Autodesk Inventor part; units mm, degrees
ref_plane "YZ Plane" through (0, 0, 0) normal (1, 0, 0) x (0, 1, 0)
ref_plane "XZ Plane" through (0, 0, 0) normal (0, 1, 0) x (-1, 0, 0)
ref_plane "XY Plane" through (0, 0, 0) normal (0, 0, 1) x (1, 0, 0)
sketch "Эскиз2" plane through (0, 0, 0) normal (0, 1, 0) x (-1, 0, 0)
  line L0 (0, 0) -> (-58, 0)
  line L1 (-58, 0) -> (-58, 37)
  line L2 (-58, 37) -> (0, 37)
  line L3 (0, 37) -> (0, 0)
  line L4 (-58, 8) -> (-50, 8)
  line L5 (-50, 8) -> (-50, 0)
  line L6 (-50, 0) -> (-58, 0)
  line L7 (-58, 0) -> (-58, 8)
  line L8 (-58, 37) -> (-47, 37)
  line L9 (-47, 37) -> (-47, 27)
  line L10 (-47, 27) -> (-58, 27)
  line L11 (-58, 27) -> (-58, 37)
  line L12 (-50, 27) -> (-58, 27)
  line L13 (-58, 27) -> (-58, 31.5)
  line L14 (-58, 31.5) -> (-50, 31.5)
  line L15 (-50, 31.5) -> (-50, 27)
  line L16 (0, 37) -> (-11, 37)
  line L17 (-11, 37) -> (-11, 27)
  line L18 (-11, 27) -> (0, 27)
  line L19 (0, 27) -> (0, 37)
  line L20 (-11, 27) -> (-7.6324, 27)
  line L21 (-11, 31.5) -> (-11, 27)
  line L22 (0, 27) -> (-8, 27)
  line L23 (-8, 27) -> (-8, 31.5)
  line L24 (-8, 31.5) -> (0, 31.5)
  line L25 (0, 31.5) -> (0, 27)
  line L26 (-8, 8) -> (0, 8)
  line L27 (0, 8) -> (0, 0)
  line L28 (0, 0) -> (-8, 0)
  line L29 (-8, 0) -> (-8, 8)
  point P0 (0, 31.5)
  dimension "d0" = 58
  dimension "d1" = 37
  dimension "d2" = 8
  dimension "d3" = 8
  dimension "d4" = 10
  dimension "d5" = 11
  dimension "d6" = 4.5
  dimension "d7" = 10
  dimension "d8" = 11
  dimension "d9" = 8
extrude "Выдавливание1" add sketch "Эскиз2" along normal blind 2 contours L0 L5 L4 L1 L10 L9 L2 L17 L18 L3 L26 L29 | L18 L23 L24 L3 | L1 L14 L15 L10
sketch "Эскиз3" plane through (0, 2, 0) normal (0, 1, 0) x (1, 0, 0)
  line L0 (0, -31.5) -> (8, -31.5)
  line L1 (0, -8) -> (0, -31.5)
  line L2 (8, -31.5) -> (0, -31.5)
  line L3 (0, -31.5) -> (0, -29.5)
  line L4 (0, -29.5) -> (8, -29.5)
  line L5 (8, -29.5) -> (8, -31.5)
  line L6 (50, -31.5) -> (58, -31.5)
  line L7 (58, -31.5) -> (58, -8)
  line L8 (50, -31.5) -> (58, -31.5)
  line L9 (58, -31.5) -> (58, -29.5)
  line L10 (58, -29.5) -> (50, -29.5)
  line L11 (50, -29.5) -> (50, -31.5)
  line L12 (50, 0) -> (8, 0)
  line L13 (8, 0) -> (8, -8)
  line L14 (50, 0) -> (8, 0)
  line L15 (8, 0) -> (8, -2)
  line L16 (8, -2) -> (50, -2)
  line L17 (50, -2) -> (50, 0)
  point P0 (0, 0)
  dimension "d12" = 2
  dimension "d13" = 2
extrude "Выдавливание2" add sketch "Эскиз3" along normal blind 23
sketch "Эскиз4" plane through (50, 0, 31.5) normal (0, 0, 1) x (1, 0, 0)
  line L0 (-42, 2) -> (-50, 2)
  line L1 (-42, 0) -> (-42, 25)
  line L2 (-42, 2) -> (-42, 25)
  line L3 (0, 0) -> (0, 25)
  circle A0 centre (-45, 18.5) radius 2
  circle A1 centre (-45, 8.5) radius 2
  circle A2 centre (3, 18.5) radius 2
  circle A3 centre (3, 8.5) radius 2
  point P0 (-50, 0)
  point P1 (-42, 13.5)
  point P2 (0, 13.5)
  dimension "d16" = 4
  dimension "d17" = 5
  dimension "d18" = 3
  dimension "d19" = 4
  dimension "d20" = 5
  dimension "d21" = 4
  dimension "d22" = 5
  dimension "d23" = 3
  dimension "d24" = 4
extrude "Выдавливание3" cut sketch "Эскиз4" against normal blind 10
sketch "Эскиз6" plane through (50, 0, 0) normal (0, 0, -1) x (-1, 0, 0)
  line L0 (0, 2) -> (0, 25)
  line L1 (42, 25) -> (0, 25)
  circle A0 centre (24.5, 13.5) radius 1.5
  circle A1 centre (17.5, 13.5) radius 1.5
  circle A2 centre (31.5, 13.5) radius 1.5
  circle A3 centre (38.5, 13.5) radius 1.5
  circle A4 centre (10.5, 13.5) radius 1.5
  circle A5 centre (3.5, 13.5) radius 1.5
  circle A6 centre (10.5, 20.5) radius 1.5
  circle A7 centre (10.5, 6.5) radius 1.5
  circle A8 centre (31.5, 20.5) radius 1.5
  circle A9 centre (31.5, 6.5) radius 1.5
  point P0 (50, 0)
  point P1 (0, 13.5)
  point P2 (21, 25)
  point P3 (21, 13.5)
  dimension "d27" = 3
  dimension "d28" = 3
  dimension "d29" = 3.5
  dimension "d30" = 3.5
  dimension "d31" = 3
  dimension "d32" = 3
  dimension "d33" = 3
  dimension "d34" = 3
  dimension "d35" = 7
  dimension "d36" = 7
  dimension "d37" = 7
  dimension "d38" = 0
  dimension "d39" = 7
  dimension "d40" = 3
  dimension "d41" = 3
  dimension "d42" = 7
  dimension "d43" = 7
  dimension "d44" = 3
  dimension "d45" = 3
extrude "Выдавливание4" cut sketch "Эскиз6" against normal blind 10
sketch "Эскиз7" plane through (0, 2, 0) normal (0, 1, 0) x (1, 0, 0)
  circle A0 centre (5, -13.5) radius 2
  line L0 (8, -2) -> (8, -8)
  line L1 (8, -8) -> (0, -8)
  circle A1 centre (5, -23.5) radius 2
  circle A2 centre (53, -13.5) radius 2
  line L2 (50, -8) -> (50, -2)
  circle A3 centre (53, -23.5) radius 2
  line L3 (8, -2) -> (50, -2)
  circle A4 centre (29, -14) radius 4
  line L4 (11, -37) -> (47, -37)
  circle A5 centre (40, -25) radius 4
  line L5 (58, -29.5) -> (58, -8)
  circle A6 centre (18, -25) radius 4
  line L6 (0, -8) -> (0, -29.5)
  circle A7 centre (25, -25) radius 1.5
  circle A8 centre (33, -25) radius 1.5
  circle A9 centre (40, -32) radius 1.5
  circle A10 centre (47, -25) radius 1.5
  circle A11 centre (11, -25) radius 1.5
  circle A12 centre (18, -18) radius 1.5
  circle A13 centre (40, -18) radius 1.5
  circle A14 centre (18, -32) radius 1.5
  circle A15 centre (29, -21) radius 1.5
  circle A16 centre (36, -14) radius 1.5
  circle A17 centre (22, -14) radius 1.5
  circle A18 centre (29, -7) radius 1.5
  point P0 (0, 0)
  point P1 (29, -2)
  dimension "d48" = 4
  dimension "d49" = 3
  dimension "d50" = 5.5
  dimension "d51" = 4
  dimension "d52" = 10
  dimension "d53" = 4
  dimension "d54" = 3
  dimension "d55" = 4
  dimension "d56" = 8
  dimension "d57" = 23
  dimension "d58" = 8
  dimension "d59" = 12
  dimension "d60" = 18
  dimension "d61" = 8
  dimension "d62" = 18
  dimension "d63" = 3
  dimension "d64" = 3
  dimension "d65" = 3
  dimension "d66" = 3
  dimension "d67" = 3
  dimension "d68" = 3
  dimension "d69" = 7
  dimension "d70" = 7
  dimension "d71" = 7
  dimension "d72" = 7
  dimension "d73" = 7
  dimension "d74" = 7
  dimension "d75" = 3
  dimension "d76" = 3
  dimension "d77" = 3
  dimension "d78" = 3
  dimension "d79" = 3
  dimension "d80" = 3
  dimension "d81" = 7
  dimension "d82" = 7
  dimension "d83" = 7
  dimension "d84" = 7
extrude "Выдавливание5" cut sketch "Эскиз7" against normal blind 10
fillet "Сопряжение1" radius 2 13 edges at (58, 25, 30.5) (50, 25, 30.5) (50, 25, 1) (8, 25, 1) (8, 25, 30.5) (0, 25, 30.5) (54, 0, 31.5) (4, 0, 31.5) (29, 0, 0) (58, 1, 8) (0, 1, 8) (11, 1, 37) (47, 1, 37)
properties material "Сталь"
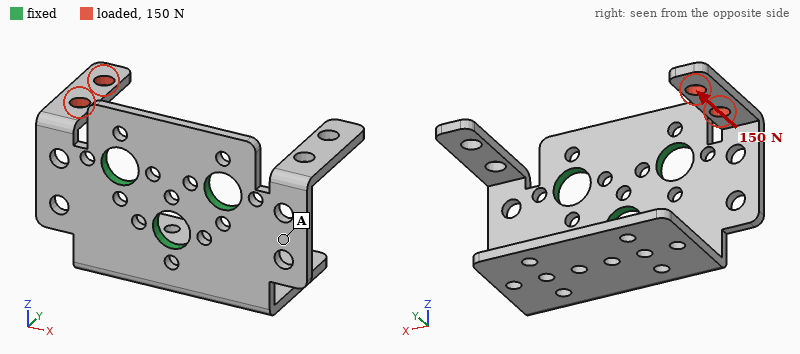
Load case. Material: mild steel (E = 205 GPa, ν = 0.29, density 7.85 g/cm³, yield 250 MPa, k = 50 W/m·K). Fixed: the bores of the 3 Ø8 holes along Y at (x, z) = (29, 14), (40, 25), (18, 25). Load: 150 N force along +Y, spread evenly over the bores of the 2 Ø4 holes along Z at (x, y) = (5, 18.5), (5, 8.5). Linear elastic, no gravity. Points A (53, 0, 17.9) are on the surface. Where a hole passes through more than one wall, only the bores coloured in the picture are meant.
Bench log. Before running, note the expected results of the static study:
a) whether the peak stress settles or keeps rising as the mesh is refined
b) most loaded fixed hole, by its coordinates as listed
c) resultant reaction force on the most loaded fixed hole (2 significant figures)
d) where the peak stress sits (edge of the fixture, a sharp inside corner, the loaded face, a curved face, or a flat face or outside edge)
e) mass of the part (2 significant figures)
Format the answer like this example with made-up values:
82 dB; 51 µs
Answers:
keeps rising; (18, 25); 180 N; a sharp inside corner; 43 g
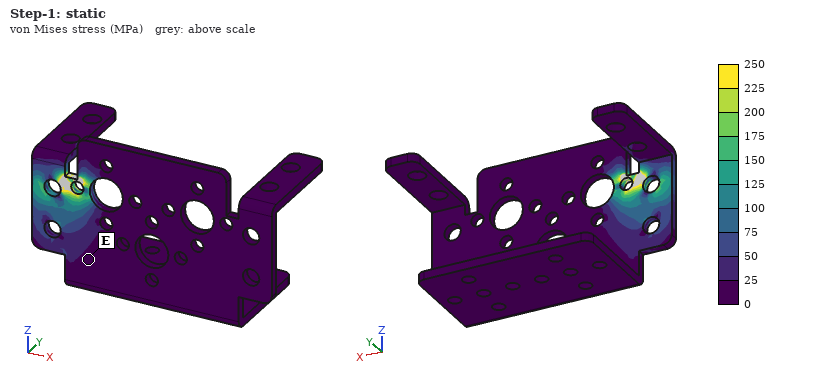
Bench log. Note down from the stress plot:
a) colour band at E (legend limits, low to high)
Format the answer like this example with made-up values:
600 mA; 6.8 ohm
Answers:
0 to 25 MPa
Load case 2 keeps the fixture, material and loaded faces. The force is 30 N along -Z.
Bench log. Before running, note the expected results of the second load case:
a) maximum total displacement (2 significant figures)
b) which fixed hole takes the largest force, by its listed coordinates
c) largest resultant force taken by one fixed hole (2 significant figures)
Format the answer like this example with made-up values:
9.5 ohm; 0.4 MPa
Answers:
0.15 mm; (18, 25); 35 N
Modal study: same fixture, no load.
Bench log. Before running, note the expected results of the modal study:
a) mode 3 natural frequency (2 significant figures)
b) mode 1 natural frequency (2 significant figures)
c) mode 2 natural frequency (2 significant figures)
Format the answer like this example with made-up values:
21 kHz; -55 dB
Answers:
1700 Hz; 1600 Hz; 1600 Hz
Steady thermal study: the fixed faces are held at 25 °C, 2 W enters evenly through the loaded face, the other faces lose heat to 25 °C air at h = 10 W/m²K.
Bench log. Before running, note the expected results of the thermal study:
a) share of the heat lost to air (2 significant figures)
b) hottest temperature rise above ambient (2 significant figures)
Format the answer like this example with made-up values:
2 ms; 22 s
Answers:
18 %; 68 K
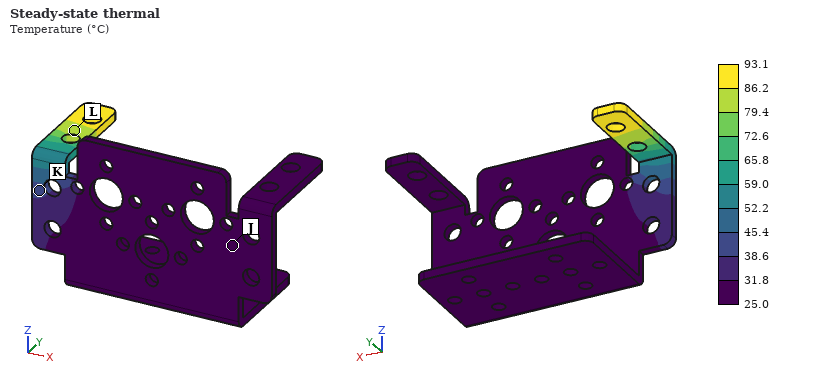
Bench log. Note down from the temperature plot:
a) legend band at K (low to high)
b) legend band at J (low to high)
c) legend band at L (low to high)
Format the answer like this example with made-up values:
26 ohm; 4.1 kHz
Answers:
38.6 to 45.4 °C; 25.0 to 31.8 °C; 79.4 to 86.2 °C
